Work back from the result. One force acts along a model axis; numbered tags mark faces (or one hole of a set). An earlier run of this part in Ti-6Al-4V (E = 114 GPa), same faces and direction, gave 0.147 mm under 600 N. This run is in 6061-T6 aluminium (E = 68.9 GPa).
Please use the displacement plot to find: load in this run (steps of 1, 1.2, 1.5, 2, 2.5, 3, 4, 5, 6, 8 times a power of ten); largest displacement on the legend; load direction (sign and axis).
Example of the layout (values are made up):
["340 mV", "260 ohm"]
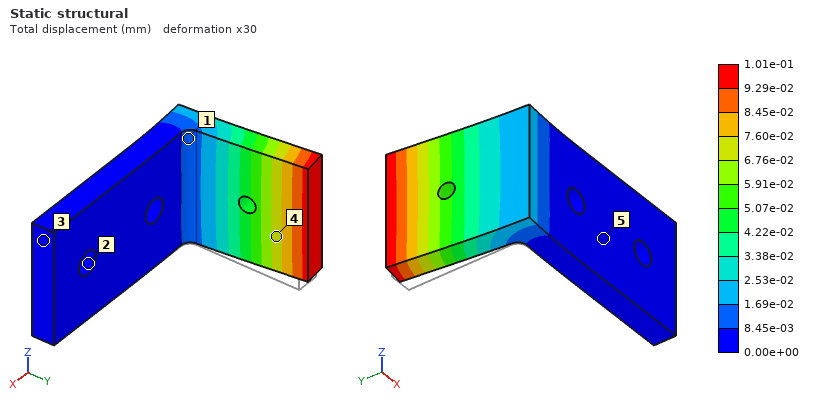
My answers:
["250 N", "1.01e-01 mm", "-X"]
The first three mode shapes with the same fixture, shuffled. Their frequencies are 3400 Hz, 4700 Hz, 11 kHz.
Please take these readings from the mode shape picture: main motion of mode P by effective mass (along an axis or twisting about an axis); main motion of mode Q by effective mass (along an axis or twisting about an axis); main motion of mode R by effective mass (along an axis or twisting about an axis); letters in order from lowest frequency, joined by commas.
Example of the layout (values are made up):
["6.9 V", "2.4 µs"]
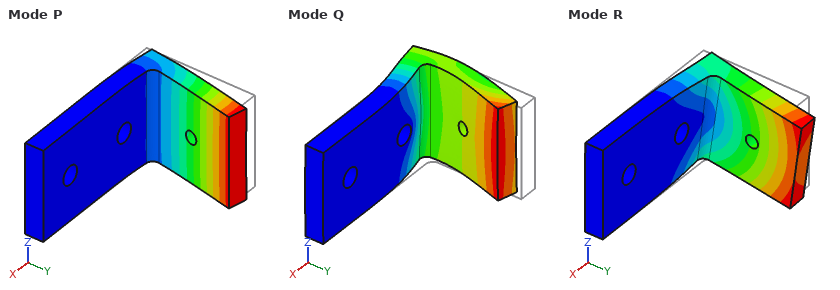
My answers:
["along X", "along Y", "along Z", "P, R, Q"]
